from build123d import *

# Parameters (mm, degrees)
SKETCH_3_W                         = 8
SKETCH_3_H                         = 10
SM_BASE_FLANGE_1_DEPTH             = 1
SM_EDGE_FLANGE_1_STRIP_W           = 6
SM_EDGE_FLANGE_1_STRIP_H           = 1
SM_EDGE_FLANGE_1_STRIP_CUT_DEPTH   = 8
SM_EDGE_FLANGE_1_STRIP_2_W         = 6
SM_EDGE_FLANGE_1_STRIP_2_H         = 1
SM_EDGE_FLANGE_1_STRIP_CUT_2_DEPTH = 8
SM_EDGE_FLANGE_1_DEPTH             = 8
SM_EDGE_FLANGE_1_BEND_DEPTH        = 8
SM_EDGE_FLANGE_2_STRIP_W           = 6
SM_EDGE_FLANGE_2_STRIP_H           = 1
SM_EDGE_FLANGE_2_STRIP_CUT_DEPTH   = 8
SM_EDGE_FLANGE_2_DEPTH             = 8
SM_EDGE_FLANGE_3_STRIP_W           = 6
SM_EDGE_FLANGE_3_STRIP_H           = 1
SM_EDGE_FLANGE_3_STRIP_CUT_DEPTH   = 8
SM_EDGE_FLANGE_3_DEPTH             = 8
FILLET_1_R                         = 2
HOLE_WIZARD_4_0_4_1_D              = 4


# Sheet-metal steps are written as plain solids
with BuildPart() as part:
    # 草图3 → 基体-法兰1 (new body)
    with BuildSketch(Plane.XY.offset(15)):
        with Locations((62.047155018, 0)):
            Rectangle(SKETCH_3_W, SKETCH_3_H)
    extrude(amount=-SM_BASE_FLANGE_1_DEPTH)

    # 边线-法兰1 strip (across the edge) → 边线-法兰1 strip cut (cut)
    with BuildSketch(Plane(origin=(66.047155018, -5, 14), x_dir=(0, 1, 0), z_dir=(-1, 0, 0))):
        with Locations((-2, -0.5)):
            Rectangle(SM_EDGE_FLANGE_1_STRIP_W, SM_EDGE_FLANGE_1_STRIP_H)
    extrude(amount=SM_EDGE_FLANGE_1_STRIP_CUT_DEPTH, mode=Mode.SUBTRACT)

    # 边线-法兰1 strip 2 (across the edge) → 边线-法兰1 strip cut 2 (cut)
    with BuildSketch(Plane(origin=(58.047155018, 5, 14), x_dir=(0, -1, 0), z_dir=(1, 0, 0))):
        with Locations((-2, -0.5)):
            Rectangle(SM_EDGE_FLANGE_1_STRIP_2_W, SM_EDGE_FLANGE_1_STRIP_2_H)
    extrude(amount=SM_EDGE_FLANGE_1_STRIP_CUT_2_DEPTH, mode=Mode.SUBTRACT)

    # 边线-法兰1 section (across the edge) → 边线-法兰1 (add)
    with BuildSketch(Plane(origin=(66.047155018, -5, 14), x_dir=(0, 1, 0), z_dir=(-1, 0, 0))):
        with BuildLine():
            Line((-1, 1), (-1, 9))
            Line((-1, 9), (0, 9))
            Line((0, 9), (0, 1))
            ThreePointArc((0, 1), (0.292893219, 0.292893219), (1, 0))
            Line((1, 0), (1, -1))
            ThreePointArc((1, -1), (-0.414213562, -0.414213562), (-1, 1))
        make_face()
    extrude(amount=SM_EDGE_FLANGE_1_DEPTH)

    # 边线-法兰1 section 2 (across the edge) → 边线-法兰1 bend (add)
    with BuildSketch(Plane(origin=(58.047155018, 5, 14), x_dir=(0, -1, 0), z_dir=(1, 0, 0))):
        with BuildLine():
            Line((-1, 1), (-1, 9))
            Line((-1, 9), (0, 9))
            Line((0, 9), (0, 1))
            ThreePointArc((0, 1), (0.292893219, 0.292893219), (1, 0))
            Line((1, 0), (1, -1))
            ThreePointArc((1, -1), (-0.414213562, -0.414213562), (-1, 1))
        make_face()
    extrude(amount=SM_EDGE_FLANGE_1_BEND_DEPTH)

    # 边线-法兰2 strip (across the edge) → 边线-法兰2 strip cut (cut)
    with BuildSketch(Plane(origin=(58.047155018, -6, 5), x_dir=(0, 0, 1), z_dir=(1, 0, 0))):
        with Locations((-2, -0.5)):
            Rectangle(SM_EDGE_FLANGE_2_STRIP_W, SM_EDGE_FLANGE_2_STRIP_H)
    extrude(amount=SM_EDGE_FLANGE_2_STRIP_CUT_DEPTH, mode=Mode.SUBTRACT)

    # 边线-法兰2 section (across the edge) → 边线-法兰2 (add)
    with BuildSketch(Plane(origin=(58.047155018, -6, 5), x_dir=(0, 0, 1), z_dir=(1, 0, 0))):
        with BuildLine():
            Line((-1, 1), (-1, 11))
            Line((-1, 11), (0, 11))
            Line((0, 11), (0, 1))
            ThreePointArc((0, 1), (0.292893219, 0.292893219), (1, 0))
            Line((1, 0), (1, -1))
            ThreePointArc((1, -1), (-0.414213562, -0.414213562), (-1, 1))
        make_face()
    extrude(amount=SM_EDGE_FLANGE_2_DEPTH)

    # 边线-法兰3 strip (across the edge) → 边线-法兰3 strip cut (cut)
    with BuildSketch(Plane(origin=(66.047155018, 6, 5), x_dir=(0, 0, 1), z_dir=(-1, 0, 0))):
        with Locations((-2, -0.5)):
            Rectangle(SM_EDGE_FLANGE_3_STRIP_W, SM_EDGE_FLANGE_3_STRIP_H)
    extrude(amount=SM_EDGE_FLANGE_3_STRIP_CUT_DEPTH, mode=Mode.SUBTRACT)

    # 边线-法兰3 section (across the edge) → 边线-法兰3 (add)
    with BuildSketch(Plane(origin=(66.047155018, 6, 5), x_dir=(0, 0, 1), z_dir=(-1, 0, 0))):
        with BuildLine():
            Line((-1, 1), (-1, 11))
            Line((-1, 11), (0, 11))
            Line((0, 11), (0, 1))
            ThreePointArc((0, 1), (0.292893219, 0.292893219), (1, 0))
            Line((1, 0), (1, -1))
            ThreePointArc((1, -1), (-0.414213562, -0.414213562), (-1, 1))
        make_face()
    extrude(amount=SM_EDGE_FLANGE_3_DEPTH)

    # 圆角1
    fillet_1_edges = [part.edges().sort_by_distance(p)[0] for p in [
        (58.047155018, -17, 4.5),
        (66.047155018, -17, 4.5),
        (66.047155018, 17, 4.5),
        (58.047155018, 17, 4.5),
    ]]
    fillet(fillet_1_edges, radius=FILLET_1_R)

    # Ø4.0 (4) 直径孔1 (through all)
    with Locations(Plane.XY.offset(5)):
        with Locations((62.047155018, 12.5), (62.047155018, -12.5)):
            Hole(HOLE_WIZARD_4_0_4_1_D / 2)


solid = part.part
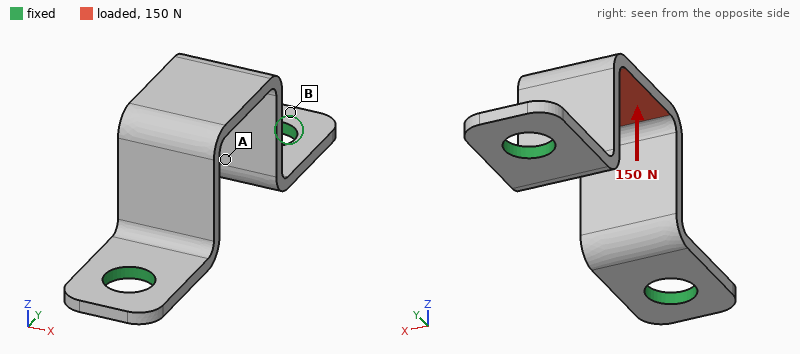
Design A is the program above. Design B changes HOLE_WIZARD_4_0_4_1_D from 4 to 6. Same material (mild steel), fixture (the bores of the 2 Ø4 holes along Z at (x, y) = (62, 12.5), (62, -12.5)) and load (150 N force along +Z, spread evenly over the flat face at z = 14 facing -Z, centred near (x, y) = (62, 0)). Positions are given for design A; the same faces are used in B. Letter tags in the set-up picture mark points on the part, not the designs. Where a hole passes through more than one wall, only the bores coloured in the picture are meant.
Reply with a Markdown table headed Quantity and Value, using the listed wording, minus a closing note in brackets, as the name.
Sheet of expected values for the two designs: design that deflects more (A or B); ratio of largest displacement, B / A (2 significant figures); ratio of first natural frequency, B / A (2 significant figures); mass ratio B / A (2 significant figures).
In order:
| Quantity | Value |
|---|---|
| design that deflects more | A |
| ratio of largest displacement, B / A | 0.76 |
| ratio of first natural frequency, B / A | 1.2 |
| mass ratio B / A | 0.92 |
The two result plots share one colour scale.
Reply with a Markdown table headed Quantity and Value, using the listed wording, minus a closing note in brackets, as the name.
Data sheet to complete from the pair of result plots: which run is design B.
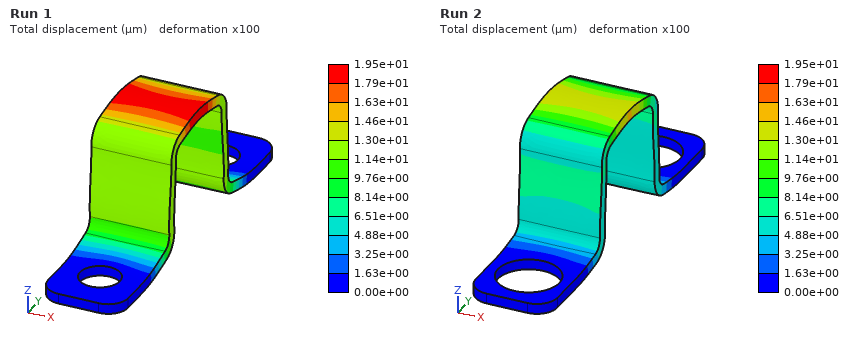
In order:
| Quantity | Value |
|---|---|
| which run is design B | Run 2 |
